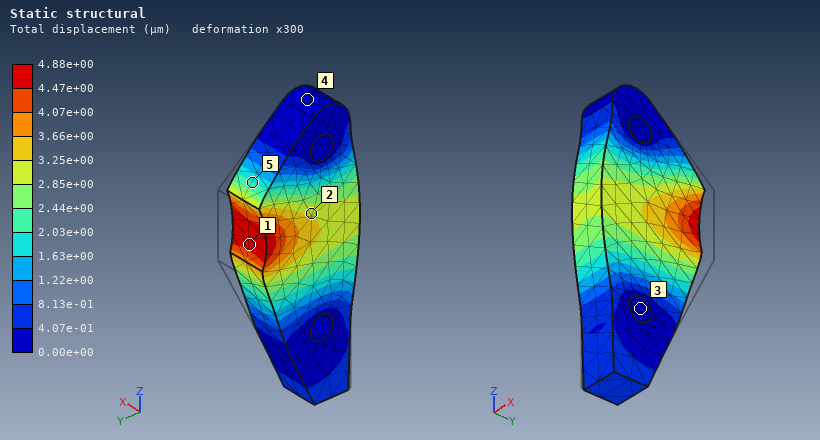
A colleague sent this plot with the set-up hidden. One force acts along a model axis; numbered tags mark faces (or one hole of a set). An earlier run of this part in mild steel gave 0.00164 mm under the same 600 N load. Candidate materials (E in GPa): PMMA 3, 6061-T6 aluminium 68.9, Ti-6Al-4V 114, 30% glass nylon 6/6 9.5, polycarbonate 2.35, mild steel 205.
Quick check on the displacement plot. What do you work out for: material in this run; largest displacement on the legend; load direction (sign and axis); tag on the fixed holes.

6061-T6 aluminium
4.88e+00 µm
-Y
3
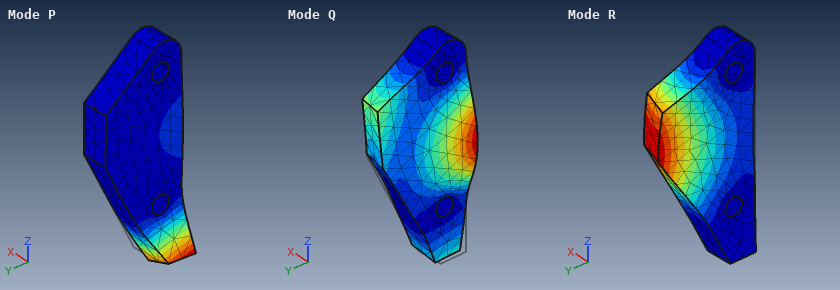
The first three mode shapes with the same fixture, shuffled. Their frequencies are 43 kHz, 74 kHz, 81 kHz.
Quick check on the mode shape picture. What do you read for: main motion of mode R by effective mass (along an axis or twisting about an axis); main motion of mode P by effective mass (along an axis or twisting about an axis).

along X
along X
